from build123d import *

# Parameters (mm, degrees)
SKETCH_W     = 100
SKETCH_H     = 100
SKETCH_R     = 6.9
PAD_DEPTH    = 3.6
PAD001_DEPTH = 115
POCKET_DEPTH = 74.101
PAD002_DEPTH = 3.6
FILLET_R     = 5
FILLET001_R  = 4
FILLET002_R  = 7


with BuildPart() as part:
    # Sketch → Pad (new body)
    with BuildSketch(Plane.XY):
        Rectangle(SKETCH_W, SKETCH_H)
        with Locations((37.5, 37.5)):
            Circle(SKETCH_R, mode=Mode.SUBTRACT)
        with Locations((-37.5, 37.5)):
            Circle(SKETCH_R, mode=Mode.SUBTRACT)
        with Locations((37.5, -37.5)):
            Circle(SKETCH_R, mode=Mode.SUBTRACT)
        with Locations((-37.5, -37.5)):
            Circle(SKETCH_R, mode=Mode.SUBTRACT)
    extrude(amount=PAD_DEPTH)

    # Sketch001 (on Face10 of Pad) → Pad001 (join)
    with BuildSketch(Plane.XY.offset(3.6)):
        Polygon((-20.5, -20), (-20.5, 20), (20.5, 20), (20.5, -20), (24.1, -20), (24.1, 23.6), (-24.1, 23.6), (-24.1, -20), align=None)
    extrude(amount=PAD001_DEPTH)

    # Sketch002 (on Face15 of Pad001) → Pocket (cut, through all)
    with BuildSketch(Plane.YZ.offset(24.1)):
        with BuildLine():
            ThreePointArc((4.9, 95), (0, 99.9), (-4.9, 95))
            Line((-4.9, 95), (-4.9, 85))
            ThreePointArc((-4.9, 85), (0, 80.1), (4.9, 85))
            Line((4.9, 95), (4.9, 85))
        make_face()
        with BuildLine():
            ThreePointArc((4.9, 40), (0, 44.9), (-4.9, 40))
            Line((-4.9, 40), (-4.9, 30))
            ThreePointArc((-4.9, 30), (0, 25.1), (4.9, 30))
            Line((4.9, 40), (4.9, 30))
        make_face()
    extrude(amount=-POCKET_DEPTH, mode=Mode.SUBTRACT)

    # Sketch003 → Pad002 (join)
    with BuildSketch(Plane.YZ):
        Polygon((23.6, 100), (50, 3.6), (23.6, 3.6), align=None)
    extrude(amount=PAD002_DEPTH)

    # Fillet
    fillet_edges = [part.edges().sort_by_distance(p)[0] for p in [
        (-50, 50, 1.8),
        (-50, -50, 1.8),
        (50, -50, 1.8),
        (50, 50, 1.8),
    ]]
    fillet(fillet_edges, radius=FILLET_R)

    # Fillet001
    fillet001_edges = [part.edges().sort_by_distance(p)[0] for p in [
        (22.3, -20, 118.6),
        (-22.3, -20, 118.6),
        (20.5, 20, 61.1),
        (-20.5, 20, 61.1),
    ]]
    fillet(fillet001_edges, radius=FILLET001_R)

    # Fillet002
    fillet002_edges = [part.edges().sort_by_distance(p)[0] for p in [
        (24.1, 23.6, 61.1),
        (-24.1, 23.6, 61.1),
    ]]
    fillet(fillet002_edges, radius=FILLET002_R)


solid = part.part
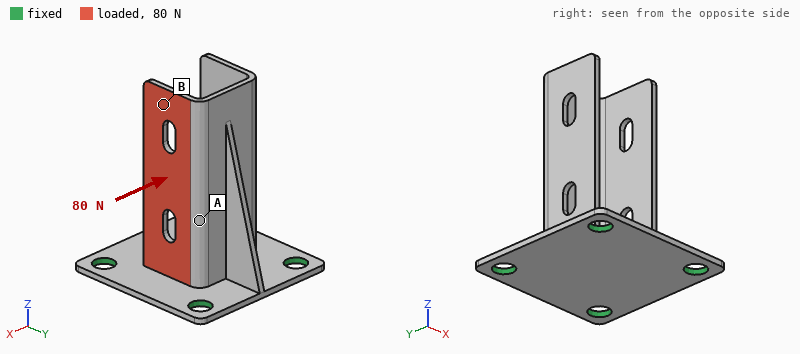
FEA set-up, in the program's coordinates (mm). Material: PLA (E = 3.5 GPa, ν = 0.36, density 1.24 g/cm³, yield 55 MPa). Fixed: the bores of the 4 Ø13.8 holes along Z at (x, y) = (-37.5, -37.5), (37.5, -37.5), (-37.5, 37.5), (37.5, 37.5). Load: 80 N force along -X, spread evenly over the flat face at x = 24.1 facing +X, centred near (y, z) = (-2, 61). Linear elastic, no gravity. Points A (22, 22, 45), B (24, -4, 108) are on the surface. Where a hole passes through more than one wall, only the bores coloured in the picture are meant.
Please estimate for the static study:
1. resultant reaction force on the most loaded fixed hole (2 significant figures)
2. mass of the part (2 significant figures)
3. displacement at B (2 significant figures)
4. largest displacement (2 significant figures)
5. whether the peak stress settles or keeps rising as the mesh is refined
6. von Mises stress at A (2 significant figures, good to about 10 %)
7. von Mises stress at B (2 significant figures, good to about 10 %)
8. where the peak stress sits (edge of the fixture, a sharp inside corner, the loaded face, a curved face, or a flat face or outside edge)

84 N
110 g
1.5 mm
2.2 mm
keeps rising
3.0 MPa
0.99 MPa
edge of the fixture
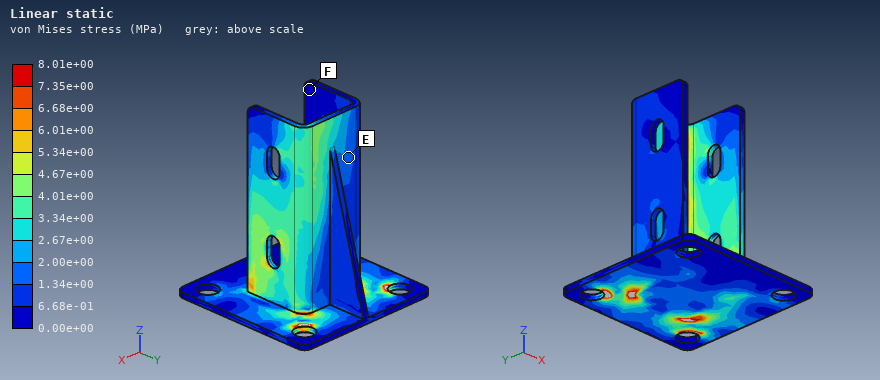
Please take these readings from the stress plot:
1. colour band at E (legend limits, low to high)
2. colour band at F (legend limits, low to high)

1.34e+00 to 2.00e+00 MPa
0.00e+00 to 6.68e-01 MPa
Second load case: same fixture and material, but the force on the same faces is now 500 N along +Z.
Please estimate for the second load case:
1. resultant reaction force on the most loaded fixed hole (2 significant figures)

240 N
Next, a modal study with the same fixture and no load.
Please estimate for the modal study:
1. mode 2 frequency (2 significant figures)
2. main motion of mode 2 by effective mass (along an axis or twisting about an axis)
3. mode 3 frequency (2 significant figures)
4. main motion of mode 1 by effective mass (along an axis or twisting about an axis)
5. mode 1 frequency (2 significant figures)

340 Hz
along Y
420 Hz
along X
220 Hz
